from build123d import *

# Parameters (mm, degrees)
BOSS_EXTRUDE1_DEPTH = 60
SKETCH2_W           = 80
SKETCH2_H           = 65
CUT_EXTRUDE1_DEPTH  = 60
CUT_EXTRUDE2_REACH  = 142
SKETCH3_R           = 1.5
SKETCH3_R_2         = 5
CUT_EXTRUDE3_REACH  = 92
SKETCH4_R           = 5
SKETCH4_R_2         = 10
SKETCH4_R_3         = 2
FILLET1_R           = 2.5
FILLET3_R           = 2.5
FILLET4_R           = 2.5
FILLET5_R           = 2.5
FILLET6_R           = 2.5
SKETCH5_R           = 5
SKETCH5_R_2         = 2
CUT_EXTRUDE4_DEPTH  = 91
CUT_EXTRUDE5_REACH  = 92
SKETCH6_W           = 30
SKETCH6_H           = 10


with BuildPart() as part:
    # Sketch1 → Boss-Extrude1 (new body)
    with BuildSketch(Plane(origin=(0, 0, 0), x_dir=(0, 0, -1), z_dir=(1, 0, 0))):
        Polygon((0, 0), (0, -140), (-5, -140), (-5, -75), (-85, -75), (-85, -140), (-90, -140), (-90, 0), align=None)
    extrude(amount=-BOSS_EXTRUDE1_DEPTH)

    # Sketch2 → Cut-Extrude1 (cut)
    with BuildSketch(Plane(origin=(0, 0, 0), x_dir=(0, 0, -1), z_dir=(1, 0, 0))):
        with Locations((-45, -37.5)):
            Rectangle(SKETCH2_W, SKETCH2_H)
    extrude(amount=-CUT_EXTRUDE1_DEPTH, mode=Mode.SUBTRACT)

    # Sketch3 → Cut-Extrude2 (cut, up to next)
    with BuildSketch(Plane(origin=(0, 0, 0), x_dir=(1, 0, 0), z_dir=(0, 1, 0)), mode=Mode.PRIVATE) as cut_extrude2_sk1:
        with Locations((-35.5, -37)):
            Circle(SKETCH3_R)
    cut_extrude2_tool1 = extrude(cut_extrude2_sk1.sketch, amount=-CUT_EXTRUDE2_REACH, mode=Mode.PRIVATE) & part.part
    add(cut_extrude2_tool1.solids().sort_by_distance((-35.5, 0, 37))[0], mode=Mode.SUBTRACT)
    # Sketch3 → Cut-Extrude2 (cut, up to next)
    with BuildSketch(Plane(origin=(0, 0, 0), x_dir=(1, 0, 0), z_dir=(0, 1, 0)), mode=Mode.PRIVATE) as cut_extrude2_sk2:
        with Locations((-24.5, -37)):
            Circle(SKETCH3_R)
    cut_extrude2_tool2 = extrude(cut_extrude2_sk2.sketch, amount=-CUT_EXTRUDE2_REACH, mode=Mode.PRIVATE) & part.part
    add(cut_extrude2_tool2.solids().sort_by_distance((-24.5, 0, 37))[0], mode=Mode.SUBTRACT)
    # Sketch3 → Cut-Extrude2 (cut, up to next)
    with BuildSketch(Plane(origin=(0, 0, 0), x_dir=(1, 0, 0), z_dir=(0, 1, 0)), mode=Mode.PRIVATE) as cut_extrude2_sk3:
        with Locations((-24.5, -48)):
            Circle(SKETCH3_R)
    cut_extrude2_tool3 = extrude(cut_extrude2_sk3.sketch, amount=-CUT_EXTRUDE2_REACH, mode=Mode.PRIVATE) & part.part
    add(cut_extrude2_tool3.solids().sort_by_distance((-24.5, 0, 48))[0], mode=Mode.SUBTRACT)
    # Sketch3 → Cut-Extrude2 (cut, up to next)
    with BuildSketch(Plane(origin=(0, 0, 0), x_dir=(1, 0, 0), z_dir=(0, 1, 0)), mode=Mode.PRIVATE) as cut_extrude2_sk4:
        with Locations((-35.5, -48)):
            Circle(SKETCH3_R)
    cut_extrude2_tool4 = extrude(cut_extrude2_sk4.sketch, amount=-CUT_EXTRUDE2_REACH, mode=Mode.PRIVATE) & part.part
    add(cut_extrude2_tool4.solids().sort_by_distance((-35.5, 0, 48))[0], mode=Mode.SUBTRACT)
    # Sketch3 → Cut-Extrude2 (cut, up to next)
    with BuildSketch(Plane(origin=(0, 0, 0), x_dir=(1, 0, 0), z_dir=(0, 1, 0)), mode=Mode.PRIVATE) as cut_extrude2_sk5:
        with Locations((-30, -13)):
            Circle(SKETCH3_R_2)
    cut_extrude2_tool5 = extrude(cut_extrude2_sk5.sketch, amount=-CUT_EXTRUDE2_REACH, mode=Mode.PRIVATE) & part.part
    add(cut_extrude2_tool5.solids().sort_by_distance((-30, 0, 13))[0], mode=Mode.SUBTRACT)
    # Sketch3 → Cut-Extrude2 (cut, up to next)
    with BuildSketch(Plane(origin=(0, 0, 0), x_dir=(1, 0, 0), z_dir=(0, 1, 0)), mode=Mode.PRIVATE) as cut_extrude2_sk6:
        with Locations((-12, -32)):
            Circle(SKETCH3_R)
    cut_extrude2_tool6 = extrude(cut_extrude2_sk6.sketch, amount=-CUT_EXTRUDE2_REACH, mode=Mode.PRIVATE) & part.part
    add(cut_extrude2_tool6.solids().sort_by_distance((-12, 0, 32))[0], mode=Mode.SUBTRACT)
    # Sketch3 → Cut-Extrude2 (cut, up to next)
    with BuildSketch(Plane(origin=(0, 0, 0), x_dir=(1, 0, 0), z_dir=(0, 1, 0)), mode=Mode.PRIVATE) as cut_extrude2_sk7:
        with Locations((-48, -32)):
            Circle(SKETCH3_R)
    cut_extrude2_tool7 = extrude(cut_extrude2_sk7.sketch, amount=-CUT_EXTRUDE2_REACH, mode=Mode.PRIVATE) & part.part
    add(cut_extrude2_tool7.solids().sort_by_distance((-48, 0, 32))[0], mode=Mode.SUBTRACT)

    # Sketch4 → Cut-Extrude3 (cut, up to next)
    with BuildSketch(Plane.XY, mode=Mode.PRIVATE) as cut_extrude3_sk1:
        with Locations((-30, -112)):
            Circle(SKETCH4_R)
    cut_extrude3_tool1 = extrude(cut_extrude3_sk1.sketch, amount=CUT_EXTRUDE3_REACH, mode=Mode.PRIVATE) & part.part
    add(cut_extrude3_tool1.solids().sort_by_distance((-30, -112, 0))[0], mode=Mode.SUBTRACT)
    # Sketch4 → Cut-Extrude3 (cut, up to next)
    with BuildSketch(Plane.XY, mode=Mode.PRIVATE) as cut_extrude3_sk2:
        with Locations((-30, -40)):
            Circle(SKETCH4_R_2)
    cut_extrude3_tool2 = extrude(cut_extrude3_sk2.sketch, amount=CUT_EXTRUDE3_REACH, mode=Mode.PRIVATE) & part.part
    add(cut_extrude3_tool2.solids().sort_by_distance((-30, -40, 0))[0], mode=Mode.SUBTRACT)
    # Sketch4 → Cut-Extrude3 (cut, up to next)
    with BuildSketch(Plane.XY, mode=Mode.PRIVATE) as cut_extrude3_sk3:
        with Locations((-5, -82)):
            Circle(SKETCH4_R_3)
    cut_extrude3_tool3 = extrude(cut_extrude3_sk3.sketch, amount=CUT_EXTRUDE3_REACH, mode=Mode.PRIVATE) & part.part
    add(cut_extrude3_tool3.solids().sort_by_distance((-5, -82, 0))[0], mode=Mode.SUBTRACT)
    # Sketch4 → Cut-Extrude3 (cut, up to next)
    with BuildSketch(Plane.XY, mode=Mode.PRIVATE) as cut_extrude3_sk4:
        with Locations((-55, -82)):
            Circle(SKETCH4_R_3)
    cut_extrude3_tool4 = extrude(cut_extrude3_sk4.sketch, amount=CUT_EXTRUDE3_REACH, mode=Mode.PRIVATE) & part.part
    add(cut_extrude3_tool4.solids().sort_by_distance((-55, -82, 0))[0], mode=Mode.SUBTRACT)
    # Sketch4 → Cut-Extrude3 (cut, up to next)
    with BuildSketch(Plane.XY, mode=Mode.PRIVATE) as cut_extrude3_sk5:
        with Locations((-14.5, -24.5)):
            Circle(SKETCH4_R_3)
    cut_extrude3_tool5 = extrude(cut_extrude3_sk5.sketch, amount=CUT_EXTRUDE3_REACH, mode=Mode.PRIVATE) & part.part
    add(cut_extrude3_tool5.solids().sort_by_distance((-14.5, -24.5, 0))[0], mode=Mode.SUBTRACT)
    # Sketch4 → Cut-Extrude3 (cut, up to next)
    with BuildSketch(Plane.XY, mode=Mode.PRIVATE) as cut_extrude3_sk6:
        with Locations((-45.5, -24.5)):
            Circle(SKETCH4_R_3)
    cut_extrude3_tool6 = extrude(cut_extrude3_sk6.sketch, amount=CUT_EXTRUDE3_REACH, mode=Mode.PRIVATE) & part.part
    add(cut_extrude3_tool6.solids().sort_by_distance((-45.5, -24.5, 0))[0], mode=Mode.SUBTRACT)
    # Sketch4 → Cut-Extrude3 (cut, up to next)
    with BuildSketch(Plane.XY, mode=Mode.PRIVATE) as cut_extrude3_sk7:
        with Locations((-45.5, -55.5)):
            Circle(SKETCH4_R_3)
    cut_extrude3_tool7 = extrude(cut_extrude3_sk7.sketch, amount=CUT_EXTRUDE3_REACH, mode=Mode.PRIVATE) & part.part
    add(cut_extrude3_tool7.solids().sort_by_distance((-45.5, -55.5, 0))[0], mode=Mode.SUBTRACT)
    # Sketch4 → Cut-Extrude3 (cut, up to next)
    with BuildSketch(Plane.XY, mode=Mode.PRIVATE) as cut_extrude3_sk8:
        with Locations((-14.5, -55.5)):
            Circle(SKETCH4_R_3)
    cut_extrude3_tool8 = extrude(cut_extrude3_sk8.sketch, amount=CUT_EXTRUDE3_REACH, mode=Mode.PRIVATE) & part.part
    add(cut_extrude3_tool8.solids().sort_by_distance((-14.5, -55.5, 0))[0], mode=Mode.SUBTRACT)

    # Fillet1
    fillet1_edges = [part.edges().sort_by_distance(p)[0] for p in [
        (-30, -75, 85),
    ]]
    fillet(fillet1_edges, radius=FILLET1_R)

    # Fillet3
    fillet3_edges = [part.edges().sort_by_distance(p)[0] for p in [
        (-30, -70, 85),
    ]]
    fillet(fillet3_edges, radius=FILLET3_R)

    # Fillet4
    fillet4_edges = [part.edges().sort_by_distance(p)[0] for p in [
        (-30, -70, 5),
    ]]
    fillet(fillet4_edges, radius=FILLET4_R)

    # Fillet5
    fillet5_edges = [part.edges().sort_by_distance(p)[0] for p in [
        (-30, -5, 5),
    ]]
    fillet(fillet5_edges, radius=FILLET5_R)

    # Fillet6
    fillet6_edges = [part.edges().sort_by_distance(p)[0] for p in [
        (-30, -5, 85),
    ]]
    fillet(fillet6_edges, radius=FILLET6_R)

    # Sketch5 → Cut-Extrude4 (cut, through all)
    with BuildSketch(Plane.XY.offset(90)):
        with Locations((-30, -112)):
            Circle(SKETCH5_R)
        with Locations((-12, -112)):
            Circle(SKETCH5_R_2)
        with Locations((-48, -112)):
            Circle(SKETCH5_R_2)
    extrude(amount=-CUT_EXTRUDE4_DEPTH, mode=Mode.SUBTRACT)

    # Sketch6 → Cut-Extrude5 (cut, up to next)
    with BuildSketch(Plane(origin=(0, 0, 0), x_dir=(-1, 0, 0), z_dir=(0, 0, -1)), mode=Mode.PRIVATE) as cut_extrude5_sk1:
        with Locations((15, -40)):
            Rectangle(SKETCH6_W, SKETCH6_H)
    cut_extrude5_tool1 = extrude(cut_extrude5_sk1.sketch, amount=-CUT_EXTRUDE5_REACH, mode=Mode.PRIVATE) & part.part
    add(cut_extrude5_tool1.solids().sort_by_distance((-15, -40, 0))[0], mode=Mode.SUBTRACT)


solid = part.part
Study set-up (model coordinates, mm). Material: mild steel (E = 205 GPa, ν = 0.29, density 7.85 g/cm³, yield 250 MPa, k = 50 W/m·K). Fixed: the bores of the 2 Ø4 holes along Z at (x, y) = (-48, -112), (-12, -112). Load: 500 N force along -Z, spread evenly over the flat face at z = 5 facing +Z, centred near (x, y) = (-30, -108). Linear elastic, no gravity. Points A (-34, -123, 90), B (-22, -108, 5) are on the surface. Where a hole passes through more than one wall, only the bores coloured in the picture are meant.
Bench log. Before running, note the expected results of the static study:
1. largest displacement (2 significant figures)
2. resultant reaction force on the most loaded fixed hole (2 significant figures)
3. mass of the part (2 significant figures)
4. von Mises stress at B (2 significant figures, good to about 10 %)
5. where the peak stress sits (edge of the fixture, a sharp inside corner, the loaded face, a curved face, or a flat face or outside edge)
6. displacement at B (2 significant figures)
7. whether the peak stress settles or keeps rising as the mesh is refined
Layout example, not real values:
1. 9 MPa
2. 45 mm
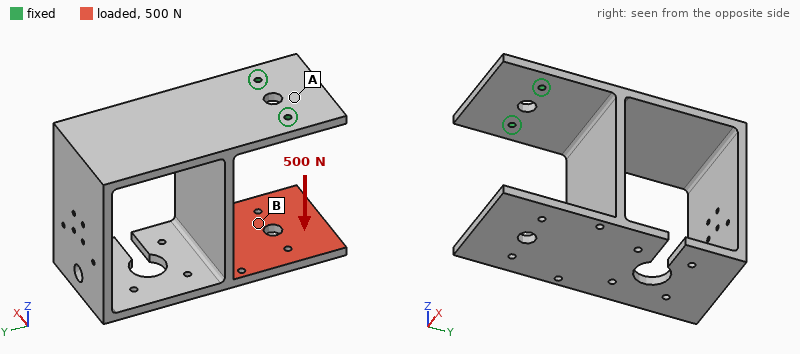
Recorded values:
1. 0.67 mm
2. 250 N
3. 1.0 kg
4. 20 MPa
5. a sharp inside corner
6. 0.41 mm
7. keeps rising
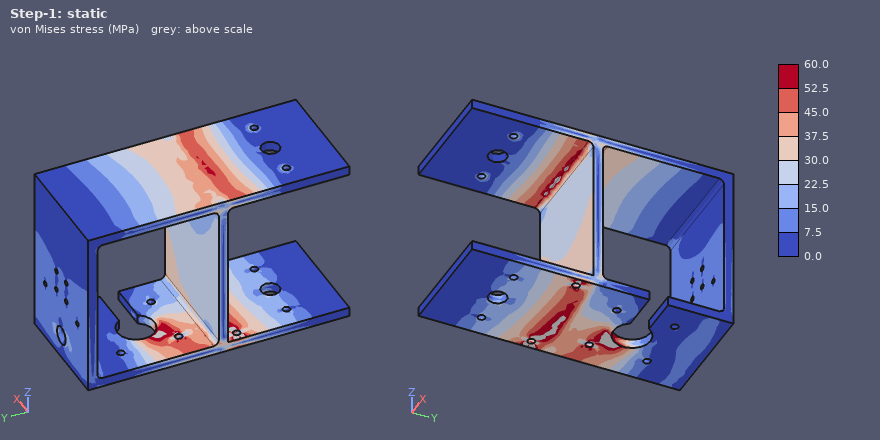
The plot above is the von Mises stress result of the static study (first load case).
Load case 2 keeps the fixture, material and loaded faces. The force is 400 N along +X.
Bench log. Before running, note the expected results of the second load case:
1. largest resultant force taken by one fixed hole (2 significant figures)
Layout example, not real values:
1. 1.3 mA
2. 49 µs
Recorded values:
1. 810 N
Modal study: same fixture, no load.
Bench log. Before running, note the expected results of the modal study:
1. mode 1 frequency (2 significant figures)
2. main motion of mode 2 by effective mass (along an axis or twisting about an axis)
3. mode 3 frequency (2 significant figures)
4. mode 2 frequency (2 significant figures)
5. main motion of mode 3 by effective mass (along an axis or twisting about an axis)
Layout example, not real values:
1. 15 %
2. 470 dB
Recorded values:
1. 110 Hz
2. along X
3. 480 Hz
4. 280 Hz
5. along Z
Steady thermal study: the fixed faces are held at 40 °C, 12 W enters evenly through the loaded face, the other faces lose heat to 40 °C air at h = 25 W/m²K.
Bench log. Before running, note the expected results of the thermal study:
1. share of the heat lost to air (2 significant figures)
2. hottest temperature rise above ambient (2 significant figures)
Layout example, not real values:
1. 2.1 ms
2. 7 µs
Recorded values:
1. 91 %
2. 38 K
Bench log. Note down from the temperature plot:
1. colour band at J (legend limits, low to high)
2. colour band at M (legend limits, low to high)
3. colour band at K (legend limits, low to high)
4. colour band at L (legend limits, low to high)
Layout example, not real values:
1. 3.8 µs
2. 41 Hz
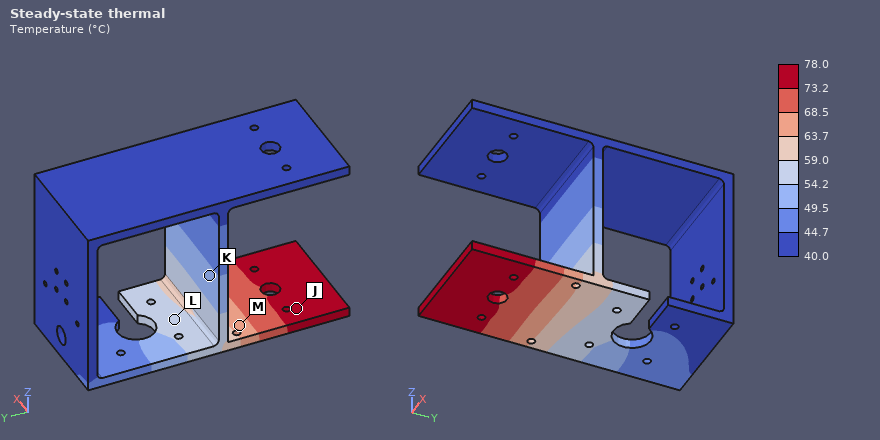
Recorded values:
1. 73.2 to 78.0 °C
2. 63.7 to 68.5 °C
3. 49.5 to 54.2 °C
4. 54.2 to 59.0 °C
